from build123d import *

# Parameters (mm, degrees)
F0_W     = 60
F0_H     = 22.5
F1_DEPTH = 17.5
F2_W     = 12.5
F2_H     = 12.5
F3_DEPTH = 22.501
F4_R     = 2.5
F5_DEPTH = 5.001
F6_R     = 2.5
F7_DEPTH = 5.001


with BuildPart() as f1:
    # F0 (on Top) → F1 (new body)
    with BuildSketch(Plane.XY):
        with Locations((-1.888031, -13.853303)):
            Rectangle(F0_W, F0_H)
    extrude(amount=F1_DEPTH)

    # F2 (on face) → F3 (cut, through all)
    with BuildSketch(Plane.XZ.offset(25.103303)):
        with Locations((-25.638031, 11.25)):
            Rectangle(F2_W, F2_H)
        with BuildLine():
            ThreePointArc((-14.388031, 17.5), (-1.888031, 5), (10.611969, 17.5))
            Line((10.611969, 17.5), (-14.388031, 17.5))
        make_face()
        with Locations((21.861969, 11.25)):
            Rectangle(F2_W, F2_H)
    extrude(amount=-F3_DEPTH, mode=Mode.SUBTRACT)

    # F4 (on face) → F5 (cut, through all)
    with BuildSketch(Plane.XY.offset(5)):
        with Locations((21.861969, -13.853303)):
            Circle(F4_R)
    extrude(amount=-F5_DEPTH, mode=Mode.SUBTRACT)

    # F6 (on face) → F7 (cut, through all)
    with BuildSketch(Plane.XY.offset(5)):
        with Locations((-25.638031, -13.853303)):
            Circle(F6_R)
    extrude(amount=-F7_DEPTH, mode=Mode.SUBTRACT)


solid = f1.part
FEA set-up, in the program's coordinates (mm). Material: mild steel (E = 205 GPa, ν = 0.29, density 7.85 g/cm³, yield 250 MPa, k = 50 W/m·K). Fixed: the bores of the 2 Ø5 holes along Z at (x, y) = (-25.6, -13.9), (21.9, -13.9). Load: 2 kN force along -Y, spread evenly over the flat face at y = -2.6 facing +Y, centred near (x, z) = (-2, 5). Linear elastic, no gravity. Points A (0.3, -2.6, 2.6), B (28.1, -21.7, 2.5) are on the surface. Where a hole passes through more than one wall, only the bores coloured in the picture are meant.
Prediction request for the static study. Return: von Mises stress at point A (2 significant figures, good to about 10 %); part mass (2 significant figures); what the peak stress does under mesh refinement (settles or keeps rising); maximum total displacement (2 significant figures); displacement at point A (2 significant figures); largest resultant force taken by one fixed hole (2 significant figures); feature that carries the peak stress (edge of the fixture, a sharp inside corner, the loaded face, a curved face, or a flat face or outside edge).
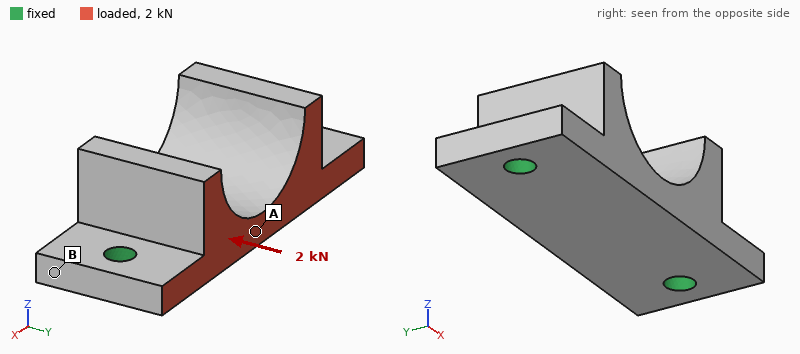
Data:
14 MPa
85 g
keeps rising
6.8 µm
3.7 µm
1.0 kN
edge of the fixture
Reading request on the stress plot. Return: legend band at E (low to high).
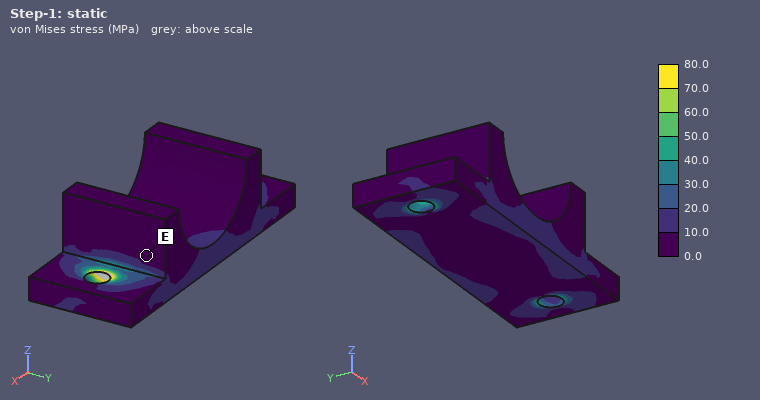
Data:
0.0 to 10.0 MPa
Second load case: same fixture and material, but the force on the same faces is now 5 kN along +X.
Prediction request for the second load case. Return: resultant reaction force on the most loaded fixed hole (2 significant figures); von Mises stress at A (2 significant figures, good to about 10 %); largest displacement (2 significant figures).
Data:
2.7 kN
20 MPa
8.3 µm
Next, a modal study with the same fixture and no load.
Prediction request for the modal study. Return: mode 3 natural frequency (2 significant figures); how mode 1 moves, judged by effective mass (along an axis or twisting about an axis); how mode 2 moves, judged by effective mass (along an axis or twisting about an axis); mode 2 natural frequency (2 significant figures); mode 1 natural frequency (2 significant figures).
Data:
16 kHz
along Z
along Y
9600 Hz
8600 Hz
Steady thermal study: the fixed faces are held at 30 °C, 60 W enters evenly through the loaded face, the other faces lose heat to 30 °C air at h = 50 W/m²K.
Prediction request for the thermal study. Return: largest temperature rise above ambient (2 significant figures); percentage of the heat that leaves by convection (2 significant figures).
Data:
66 K
12 %
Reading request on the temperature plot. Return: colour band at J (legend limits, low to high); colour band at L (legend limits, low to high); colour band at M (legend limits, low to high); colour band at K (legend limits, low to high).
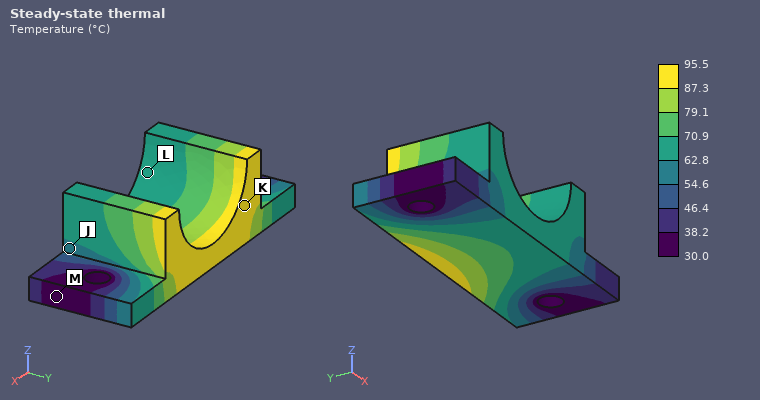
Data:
54.6 to 62.8 °C
62.8 to 70.9 °C
30.0 to 38.2 °C
87.3 to 95.5 °C
